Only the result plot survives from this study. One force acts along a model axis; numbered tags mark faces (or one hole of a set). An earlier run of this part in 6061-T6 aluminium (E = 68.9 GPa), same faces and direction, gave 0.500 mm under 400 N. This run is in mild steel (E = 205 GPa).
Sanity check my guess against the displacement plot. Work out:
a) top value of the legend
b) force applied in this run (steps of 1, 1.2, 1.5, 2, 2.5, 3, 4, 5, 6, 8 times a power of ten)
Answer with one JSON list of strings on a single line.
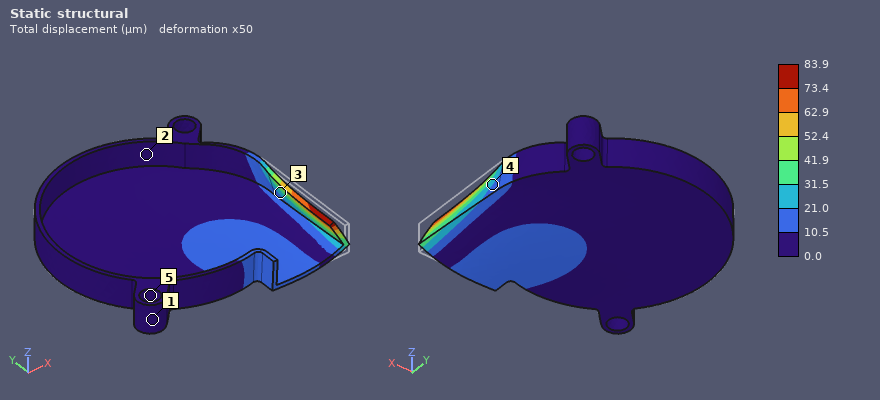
["83.9 µm", "200 N"]
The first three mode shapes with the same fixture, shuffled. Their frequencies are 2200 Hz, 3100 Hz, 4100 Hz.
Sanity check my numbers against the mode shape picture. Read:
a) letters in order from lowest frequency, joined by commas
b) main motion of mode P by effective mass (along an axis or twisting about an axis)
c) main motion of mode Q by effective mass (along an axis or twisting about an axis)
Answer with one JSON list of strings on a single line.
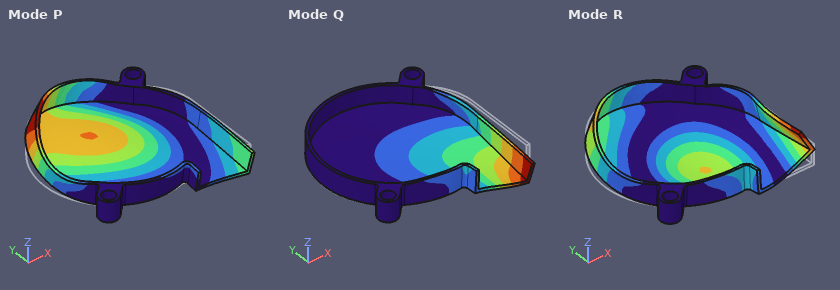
["Q, P, R", "along Z", "along Z"]
